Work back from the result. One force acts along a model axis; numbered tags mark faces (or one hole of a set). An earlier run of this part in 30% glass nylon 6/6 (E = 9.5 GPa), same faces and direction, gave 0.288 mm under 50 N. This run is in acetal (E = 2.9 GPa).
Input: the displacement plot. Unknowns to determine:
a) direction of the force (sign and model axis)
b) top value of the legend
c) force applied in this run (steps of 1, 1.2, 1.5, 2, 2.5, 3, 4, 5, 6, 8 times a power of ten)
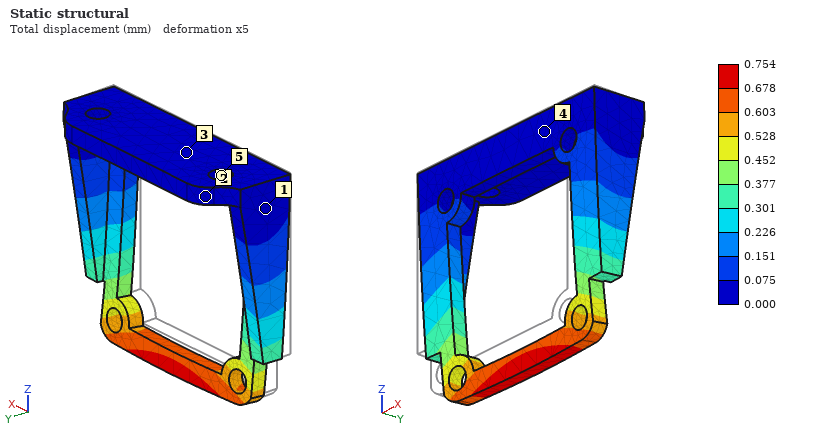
+Y
0.754 mm
40 N
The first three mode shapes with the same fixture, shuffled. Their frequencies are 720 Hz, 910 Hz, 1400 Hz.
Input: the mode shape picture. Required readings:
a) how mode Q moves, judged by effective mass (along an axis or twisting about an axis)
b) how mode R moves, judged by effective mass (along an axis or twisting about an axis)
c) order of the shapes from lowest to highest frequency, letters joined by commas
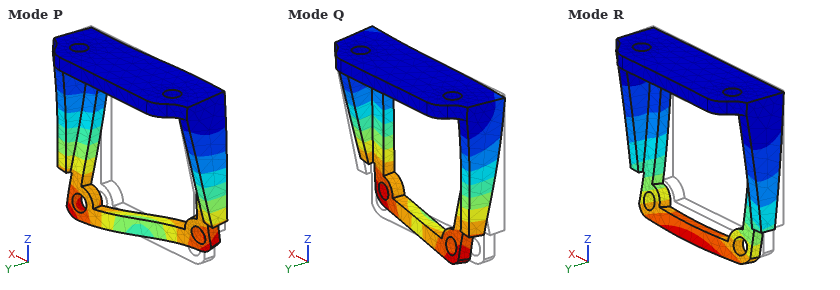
along X
along Y
R, Q, P
